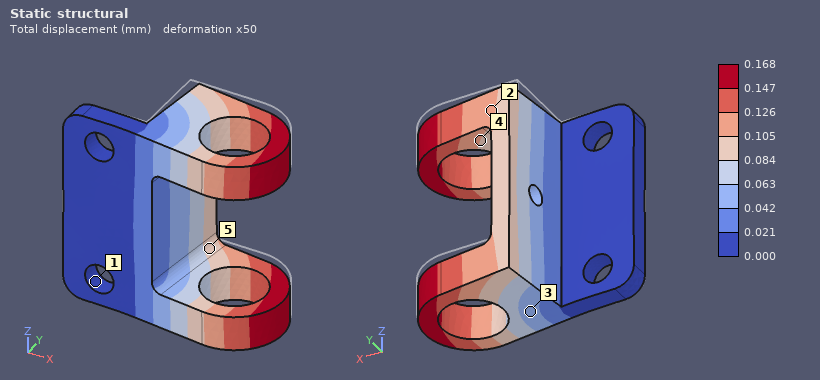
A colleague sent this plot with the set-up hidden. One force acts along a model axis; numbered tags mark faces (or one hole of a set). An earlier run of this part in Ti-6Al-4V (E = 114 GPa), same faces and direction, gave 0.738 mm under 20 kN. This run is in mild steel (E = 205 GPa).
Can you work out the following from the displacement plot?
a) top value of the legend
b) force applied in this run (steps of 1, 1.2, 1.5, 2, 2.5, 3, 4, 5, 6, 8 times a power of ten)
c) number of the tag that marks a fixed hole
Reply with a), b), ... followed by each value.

a) 0.168 mm
b) 8 kN
c) 1
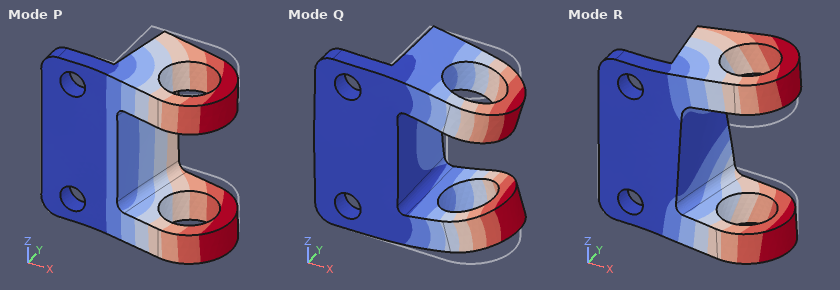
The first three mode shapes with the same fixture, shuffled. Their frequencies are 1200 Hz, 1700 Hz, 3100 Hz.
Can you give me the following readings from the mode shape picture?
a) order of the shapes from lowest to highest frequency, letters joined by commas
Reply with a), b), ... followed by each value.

a) P, R, Q
